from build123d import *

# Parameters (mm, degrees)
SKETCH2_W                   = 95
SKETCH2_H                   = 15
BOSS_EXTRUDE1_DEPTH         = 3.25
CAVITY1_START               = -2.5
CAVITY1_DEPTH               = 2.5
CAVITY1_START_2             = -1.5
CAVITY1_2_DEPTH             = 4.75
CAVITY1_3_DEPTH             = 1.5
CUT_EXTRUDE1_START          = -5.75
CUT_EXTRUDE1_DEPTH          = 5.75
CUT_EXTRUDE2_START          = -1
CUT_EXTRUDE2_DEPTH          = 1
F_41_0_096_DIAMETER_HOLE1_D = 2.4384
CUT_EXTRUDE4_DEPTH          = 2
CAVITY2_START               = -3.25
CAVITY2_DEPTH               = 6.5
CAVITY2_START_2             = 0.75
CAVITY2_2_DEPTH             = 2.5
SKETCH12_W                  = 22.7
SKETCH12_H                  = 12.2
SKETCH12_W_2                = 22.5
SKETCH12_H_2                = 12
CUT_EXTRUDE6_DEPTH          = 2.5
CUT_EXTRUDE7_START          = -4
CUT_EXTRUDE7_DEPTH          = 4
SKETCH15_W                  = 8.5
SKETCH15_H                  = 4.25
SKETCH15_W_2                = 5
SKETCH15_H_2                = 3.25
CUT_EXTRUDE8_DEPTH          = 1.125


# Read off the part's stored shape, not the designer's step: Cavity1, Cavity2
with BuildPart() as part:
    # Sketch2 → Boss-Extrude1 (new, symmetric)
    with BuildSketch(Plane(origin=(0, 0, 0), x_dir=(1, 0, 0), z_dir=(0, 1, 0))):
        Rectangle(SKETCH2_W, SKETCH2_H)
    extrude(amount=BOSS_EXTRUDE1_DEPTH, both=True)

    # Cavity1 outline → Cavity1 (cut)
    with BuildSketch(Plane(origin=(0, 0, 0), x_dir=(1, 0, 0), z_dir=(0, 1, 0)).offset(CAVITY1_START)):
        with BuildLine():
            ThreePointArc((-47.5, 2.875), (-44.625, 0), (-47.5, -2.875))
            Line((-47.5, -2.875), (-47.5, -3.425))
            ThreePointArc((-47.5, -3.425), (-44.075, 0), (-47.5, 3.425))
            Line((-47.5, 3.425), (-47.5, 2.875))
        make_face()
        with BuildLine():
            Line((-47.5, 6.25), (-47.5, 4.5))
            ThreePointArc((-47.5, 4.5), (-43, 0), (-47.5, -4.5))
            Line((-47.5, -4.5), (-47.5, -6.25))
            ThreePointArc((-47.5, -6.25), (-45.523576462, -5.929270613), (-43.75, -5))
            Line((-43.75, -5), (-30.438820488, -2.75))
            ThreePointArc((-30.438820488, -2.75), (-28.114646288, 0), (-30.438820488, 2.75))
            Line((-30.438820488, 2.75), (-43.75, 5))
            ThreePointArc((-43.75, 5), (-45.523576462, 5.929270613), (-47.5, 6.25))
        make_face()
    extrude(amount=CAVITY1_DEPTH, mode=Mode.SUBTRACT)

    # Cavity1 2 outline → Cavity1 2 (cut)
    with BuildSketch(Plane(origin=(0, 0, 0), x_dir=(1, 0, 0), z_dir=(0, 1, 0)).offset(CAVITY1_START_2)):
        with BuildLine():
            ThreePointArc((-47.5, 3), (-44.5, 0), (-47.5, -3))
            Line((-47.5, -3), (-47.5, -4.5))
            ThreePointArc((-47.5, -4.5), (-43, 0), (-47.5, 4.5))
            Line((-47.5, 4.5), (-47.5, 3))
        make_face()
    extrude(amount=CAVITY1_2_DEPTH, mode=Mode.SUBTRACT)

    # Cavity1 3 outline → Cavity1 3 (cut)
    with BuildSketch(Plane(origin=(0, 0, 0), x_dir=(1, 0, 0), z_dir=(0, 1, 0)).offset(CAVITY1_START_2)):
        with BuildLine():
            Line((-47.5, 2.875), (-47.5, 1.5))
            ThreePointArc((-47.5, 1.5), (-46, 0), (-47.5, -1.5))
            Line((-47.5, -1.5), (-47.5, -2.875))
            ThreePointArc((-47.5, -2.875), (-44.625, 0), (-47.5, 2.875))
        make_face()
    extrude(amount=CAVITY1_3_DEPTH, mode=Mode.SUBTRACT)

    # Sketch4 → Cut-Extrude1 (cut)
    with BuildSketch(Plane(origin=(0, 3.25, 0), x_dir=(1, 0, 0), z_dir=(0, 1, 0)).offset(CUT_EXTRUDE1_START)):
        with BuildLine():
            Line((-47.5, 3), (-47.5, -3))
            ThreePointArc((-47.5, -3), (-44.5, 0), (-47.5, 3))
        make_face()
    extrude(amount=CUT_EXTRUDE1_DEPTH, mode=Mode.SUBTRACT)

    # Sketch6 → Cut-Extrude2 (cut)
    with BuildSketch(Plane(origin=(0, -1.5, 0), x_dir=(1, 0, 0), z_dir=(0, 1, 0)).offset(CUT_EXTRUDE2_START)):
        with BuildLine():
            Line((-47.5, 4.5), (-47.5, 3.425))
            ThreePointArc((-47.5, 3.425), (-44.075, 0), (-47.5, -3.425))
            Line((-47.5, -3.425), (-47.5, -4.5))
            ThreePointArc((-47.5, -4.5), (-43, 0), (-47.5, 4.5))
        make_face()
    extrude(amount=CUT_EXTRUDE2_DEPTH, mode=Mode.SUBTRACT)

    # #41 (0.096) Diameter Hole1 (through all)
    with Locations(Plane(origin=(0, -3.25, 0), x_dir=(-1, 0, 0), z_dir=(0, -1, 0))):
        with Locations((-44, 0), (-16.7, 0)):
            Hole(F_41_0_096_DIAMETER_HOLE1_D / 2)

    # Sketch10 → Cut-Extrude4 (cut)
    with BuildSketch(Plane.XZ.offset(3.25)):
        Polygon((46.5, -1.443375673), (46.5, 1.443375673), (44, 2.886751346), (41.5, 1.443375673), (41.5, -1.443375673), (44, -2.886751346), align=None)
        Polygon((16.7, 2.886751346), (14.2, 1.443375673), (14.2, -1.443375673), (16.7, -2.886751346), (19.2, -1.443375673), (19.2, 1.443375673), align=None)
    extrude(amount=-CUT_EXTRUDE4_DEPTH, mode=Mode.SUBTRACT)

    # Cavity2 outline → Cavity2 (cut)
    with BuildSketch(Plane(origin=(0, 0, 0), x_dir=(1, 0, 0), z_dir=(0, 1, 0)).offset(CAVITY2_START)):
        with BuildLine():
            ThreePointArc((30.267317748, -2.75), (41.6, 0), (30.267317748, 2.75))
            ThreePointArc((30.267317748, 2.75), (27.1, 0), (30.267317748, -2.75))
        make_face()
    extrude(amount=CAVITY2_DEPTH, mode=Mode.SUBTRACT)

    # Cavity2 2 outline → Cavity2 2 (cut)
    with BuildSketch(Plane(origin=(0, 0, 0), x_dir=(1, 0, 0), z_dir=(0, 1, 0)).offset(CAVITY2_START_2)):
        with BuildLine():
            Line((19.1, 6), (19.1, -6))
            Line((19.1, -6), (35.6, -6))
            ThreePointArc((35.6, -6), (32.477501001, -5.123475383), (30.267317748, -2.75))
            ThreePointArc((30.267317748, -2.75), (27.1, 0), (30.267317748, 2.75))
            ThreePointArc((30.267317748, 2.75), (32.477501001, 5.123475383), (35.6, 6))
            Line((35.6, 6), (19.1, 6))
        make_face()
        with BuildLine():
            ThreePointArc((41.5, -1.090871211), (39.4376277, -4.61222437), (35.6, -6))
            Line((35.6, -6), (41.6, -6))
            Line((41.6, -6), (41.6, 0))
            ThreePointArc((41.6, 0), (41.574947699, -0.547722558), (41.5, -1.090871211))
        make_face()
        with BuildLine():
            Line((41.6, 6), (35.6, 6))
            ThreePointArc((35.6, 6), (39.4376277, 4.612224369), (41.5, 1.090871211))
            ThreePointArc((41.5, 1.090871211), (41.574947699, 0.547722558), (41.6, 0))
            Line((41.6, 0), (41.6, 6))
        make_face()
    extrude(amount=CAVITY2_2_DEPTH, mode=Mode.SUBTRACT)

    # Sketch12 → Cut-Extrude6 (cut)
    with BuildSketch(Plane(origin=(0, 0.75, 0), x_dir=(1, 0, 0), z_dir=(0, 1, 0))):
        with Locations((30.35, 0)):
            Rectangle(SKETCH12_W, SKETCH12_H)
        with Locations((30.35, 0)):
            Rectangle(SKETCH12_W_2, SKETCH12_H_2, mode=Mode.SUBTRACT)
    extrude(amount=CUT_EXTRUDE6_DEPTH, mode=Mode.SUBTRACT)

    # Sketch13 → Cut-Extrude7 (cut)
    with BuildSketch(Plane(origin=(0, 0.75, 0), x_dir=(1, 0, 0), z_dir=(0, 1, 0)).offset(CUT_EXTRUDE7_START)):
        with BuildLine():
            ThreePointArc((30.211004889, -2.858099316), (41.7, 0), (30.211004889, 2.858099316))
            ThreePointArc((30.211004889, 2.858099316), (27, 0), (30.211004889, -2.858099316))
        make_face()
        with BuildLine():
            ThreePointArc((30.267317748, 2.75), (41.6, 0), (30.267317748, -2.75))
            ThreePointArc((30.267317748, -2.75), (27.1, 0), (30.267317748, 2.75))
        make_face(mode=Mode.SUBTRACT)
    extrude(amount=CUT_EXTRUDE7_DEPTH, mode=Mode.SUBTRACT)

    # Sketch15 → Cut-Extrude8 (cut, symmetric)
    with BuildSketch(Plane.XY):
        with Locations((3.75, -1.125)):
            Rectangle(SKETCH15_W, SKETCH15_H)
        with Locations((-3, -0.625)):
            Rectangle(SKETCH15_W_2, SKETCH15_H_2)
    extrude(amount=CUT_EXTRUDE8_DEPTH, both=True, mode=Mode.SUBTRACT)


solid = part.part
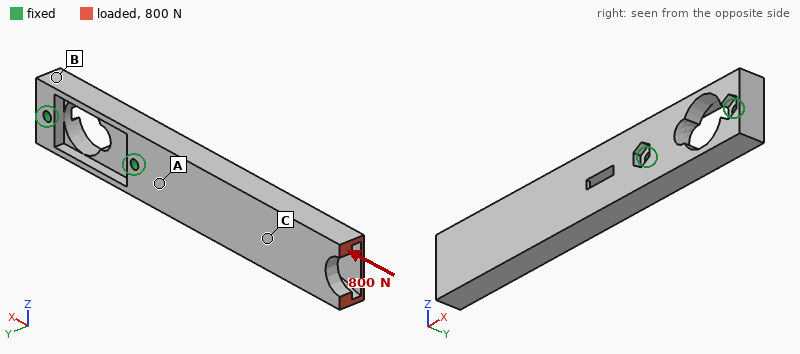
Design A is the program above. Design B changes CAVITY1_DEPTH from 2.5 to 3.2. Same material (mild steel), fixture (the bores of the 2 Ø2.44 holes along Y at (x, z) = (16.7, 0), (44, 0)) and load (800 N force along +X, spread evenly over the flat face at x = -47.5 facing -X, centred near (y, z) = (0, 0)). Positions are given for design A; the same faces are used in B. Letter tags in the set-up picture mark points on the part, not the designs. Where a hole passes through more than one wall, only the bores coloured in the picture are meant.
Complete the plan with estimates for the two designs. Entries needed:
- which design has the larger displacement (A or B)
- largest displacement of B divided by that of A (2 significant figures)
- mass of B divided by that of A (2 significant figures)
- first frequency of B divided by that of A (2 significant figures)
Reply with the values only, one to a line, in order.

B
1.1
0.99
1.0
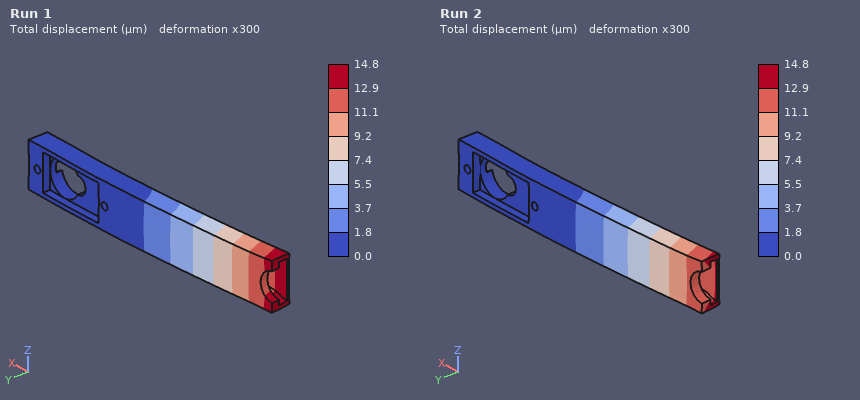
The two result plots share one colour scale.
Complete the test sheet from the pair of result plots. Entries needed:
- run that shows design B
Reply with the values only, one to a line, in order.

Run 1
